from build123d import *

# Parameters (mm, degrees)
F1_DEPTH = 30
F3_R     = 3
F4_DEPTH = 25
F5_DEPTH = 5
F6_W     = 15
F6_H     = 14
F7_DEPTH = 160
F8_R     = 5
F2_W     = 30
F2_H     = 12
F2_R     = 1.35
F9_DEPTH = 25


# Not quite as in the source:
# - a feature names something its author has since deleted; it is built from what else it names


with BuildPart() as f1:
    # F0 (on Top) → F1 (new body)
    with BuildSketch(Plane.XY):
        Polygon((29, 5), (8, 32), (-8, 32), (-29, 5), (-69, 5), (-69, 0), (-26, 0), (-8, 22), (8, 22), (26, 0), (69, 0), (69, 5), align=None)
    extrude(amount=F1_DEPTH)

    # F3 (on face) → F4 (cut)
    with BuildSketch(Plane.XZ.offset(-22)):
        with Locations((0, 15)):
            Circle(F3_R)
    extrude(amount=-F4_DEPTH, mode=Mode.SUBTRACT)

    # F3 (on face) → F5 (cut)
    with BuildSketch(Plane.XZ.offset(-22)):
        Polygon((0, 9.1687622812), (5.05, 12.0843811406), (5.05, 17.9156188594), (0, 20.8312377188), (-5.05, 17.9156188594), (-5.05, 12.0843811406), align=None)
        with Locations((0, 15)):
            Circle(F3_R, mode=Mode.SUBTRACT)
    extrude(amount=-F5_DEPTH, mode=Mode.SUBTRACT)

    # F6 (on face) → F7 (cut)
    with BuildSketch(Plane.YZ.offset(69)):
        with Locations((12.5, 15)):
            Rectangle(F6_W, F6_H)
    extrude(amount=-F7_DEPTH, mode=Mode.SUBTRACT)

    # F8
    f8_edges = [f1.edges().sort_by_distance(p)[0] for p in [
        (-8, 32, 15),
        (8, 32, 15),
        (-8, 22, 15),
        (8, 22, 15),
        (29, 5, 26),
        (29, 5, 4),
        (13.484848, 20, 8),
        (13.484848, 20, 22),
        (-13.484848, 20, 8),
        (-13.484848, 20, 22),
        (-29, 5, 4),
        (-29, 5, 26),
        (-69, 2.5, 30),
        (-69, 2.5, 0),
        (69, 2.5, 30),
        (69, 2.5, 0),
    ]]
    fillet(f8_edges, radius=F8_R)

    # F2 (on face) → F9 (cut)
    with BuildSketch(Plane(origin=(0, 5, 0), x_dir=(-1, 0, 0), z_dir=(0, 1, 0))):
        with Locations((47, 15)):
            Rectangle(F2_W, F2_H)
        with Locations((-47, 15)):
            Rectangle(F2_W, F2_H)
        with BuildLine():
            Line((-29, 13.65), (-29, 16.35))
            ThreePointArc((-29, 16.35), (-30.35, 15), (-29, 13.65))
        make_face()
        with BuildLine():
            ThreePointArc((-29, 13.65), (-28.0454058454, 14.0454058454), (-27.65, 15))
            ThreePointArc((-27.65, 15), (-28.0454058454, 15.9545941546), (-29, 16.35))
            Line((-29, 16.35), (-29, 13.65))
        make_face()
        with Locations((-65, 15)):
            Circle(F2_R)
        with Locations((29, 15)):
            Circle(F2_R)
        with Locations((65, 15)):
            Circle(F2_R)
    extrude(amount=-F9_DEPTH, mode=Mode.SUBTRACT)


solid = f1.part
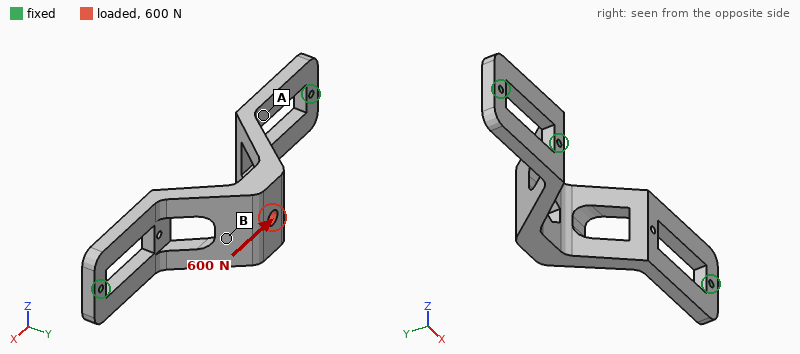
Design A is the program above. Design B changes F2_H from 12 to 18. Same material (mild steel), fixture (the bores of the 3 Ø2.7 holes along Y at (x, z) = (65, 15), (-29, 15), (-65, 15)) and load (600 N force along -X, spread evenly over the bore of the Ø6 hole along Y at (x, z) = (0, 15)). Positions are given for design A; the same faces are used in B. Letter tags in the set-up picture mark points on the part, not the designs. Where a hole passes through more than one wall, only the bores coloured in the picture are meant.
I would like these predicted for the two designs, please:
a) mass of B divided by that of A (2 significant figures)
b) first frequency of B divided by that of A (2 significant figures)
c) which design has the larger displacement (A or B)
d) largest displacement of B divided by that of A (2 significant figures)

0.91
0.91
B
1.3
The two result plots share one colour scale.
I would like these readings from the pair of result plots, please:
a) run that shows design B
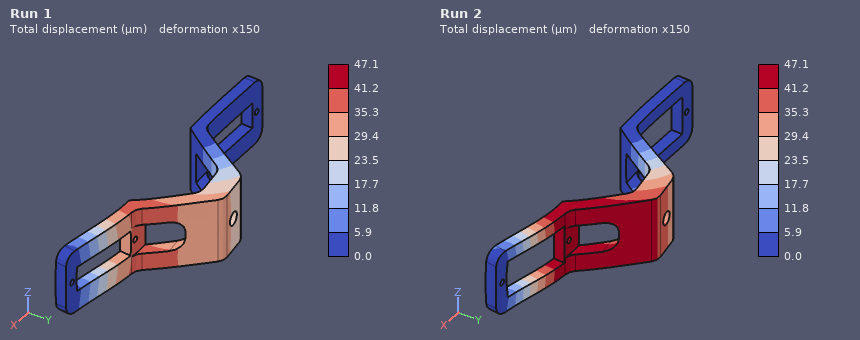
Run 2
